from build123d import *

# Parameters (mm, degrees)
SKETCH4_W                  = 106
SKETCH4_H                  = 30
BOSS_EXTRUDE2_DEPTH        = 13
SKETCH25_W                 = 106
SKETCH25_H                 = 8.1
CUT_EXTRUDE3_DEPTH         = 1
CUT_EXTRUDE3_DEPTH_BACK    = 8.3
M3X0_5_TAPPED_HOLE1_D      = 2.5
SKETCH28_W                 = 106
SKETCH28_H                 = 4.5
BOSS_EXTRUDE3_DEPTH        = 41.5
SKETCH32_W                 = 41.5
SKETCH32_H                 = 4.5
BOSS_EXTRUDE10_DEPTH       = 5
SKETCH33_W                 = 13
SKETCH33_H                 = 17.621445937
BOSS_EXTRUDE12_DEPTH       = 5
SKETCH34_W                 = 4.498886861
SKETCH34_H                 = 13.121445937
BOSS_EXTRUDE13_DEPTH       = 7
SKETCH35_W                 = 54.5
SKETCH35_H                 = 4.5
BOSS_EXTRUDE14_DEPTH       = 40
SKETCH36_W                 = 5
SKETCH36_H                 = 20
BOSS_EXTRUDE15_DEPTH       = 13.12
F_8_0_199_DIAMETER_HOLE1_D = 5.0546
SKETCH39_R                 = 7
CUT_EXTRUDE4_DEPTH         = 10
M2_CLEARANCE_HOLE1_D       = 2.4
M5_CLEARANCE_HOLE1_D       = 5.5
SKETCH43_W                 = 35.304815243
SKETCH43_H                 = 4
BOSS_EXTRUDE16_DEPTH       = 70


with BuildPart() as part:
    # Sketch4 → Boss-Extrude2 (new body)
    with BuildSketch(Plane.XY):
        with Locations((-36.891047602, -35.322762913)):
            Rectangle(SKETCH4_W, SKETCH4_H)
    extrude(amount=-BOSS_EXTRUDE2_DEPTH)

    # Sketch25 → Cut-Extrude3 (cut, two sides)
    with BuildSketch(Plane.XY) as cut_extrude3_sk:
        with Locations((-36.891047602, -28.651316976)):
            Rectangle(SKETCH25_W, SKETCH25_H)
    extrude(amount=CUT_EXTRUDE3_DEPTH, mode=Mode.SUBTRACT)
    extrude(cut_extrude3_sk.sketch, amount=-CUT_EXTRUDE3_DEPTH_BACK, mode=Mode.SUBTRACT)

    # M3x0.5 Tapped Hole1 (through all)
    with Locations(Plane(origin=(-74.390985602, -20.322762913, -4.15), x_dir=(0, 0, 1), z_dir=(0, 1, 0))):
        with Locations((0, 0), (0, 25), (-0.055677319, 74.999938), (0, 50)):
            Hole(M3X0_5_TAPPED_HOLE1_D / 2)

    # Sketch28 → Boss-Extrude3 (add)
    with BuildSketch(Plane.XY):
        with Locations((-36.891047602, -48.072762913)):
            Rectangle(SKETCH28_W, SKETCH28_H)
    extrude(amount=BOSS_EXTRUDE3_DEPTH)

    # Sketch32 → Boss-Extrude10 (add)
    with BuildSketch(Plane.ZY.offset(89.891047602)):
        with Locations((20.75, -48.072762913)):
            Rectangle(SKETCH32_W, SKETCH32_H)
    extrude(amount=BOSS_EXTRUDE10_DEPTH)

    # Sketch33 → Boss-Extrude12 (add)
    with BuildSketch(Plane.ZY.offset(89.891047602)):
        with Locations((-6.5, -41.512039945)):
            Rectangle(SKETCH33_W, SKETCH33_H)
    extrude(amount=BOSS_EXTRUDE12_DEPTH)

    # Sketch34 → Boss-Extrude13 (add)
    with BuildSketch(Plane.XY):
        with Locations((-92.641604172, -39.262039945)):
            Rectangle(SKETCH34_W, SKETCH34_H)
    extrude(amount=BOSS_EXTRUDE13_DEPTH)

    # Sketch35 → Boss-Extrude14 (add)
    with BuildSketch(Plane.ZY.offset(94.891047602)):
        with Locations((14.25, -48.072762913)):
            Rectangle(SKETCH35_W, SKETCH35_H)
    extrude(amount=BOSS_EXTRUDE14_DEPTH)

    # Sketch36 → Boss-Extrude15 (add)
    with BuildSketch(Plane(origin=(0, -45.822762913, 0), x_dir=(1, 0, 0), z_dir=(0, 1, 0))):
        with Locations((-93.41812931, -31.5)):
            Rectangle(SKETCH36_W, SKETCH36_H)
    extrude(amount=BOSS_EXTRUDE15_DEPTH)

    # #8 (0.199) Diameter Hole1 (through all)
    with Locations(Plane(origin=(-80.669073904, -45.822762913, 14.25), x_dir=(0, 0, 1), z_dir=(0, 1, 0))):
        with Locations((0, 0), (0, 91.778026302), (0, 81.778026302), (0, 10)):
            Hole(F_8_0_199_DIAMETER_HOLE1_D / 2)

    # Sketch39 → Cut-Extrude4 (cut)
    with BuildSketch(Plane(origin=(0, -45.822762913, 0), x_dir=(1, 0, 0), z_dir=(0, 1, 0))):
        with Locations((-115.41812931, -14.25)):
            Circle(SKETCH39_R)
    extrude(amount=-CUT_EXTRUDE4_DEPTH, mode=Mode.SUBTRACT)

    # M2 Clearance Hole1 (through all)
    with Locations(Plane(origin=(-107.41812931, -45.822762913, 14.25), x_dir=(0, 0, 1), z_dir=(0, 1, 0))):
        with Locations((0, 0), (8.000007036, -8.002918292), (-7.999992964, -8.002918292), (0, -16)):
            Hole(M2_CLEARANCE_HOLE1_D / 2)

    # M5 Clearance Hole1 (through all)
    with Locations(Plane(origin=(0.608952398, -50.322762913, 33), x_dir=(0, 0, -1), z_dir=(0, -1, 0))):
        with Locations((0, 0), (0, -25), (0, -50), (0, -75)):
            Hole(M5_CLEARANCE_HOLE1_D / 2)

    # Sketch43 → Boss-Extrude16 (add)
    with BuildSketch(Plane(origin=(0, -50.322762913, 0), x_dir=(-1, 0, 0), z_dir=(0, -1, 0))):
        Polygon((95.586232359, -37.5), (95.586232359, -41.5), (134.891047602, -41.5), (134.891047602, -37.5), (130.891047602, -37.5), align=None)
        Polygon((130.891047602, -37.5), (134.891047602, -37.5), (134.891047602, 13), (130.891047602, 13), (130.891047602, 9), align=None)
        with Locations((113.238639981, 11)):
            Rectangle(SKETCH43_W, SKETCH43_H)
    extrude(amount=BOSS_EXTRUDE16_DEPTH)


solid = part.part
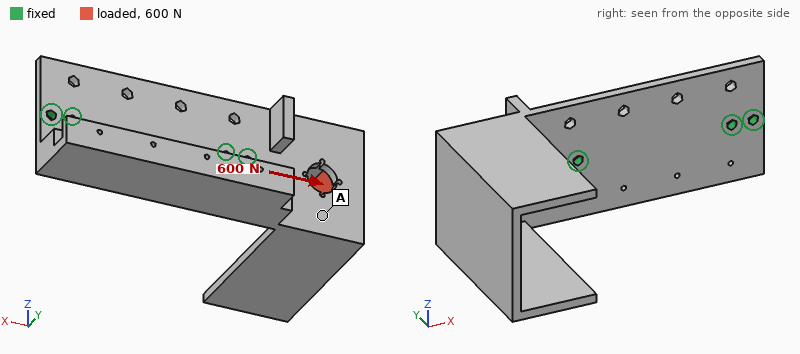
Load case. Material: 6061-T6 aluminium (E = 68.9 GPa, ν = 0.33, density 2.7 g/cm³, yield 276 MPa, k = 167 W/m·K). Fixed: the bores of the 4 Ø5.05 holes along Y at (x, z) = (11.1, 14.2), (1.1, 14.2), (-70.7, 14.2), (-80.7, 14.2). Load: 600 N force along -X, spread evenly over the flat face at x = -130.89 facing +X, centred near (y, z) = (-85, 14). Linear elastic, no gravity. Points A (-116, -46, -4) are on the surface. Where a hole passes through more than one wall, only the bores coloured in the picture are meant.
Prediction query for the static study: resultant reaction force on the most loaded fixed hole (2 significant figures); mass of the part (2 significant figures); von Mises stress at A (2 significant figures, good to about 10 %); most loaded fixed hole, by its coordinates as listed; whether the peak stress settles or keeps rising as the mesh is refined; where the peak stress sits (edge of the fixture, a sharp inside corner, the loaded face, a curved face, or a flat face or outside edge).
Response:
670 N
270 g
14 MPa
(-80.7, 14.2)
keeps rising
a sharp inside corner
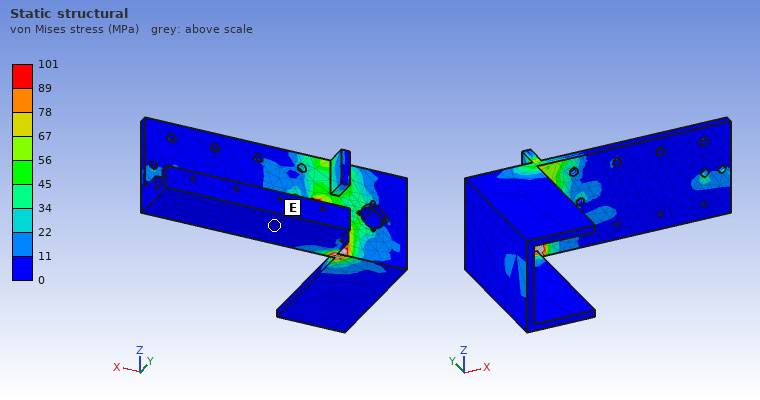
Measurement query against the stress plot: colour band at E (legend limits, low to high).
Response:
0 to 11 MPa
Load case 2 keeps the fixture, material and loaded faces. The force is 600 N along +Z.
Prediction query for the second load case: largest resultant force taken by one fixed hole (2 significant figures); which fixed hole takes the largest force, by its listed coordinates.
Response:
1.0 kN
(-80.7, 14.2)
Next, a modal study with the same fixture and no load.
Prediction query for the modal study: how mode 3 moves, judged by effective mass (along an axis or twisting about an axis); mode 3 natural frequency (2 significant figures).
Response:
along Y
1500 Hz
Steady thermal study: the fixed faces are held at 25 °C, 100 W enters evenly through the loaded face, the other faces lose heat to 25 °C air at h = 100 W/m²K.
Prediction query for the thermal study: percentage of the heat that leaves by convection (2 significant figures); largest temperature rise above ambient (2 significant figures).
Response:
77 %
56 K
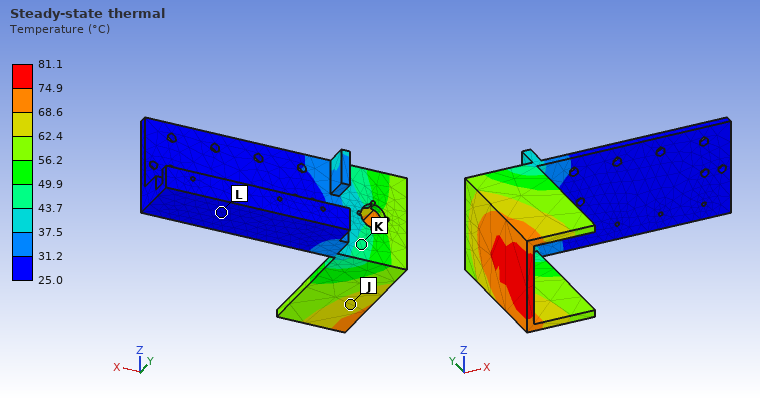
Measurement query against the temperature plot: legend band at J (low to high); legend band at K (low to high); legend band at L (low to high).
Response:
62.4 to 68.6 °C
43.7 to 49.9 °C
25.0 to 31.2 °C
